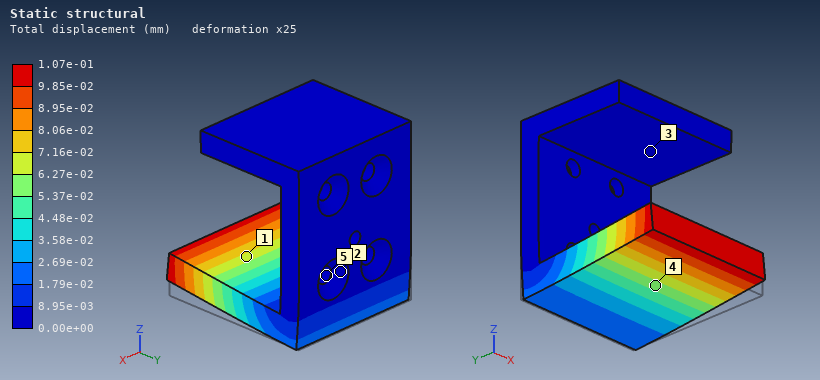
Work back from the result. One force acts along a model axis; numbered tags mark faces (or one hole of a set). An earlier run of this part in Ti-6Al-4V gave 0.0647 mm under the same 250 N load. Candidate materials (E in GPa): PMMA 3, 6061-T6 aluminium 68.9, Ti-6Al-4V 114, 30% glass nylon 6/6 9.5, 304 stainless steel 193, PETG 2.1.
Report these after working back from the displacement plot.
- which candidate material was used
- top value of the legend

6061-T6 aluminium
1.07e-01 mm
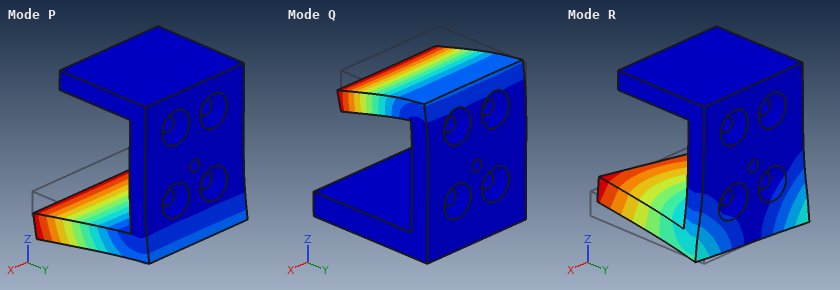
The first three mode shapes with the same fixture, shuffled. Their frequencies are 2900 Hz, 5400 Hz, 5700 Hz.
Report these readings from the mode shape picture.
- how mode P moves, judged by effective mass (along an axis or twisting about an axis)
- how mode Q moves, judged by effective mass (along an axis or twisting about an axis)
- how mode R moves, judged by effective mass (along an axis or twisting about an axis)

along Z
along Z
along X
